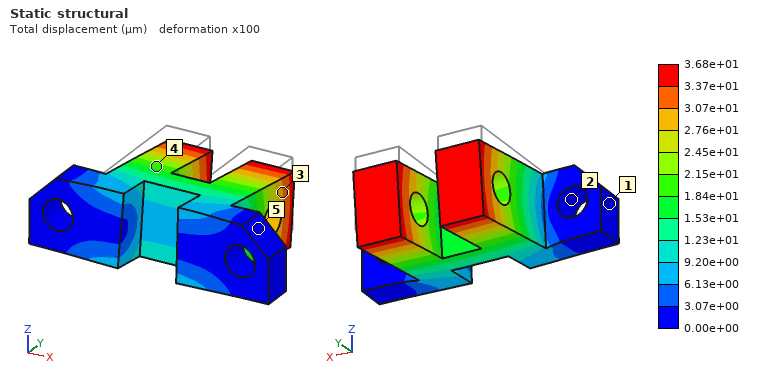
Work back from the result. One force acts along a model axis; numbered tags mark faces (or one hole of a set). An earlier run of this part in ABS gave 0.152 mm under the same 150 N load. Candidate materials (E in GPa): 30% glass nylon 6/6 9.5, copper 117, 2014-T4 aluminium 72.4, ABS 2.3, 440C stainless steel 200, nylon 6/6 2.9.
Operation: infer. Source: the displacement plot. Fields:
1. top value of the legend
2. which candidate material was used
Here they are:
3.68e+01 µm
30% glass nylon 6/6
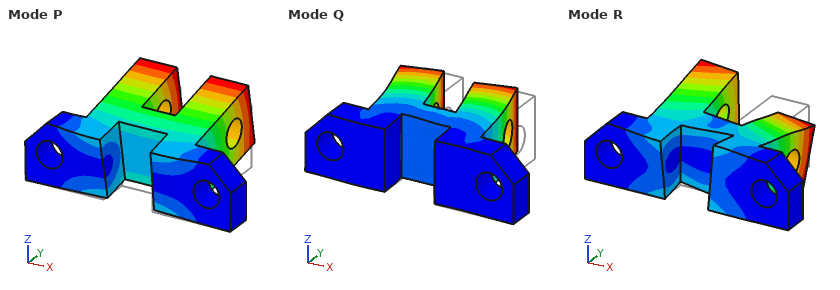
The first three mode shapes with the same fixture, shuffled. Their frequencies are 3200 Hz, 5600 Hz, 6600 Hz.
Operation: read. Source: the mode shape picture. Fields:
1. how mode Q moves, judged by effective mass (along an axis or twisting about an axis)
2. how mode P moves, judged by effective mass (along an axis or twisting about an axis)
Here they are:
along X
along Z
